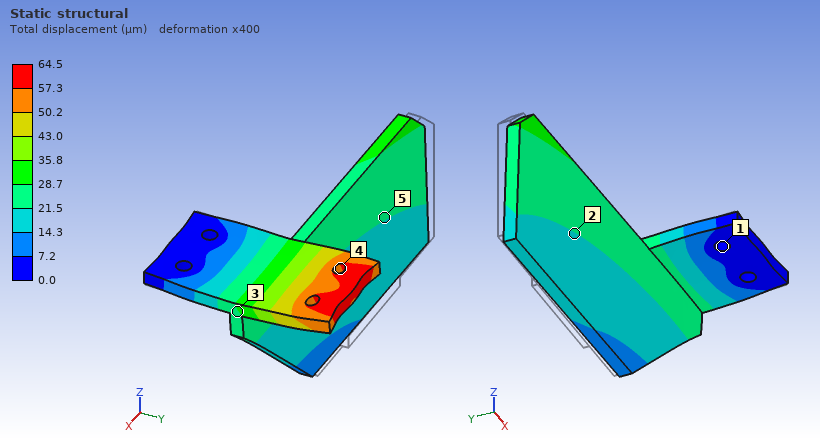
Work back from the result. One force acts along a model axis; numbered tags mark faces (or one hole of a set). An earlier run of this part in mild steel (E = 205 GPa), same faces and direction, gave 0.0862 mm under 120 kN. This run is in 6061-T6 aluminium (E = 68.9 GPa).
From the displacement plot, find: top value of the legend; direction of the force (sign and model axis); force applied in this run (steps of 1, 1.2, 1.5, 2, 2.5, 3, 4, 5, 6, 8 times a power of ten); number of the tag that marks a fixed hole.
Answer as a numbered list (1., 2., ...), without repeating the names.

1. 64.5 µm
2. -Y
3. 30 kN
4. 1
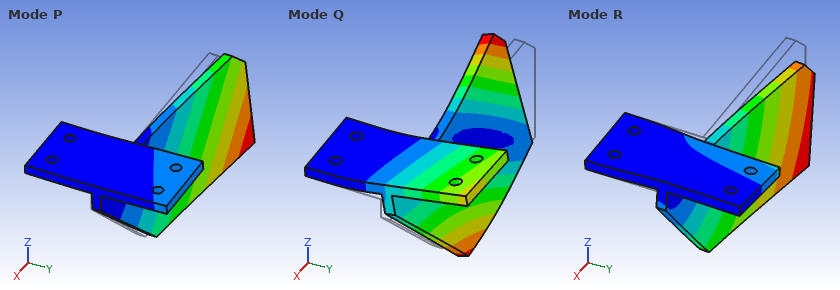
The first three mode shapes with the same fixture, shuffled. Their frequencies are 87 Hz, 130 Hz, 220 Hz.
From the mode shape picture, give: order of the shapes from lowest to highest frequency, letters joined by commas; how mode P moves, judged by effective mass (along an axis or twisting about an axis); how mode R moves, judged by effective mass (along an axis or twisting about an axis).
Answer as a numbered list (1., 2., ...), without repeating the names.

1. P, R, Q
2. along Y
3. along Z
